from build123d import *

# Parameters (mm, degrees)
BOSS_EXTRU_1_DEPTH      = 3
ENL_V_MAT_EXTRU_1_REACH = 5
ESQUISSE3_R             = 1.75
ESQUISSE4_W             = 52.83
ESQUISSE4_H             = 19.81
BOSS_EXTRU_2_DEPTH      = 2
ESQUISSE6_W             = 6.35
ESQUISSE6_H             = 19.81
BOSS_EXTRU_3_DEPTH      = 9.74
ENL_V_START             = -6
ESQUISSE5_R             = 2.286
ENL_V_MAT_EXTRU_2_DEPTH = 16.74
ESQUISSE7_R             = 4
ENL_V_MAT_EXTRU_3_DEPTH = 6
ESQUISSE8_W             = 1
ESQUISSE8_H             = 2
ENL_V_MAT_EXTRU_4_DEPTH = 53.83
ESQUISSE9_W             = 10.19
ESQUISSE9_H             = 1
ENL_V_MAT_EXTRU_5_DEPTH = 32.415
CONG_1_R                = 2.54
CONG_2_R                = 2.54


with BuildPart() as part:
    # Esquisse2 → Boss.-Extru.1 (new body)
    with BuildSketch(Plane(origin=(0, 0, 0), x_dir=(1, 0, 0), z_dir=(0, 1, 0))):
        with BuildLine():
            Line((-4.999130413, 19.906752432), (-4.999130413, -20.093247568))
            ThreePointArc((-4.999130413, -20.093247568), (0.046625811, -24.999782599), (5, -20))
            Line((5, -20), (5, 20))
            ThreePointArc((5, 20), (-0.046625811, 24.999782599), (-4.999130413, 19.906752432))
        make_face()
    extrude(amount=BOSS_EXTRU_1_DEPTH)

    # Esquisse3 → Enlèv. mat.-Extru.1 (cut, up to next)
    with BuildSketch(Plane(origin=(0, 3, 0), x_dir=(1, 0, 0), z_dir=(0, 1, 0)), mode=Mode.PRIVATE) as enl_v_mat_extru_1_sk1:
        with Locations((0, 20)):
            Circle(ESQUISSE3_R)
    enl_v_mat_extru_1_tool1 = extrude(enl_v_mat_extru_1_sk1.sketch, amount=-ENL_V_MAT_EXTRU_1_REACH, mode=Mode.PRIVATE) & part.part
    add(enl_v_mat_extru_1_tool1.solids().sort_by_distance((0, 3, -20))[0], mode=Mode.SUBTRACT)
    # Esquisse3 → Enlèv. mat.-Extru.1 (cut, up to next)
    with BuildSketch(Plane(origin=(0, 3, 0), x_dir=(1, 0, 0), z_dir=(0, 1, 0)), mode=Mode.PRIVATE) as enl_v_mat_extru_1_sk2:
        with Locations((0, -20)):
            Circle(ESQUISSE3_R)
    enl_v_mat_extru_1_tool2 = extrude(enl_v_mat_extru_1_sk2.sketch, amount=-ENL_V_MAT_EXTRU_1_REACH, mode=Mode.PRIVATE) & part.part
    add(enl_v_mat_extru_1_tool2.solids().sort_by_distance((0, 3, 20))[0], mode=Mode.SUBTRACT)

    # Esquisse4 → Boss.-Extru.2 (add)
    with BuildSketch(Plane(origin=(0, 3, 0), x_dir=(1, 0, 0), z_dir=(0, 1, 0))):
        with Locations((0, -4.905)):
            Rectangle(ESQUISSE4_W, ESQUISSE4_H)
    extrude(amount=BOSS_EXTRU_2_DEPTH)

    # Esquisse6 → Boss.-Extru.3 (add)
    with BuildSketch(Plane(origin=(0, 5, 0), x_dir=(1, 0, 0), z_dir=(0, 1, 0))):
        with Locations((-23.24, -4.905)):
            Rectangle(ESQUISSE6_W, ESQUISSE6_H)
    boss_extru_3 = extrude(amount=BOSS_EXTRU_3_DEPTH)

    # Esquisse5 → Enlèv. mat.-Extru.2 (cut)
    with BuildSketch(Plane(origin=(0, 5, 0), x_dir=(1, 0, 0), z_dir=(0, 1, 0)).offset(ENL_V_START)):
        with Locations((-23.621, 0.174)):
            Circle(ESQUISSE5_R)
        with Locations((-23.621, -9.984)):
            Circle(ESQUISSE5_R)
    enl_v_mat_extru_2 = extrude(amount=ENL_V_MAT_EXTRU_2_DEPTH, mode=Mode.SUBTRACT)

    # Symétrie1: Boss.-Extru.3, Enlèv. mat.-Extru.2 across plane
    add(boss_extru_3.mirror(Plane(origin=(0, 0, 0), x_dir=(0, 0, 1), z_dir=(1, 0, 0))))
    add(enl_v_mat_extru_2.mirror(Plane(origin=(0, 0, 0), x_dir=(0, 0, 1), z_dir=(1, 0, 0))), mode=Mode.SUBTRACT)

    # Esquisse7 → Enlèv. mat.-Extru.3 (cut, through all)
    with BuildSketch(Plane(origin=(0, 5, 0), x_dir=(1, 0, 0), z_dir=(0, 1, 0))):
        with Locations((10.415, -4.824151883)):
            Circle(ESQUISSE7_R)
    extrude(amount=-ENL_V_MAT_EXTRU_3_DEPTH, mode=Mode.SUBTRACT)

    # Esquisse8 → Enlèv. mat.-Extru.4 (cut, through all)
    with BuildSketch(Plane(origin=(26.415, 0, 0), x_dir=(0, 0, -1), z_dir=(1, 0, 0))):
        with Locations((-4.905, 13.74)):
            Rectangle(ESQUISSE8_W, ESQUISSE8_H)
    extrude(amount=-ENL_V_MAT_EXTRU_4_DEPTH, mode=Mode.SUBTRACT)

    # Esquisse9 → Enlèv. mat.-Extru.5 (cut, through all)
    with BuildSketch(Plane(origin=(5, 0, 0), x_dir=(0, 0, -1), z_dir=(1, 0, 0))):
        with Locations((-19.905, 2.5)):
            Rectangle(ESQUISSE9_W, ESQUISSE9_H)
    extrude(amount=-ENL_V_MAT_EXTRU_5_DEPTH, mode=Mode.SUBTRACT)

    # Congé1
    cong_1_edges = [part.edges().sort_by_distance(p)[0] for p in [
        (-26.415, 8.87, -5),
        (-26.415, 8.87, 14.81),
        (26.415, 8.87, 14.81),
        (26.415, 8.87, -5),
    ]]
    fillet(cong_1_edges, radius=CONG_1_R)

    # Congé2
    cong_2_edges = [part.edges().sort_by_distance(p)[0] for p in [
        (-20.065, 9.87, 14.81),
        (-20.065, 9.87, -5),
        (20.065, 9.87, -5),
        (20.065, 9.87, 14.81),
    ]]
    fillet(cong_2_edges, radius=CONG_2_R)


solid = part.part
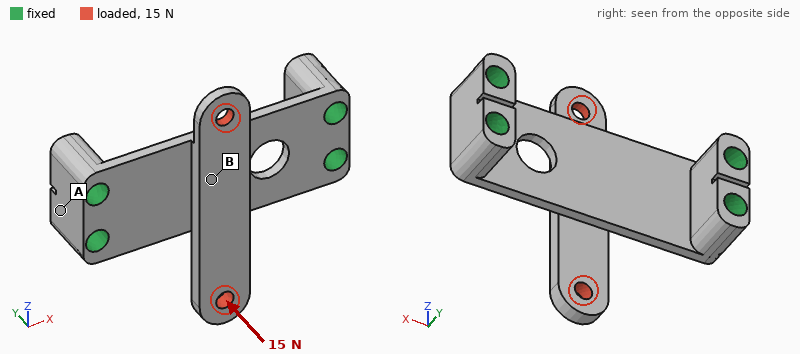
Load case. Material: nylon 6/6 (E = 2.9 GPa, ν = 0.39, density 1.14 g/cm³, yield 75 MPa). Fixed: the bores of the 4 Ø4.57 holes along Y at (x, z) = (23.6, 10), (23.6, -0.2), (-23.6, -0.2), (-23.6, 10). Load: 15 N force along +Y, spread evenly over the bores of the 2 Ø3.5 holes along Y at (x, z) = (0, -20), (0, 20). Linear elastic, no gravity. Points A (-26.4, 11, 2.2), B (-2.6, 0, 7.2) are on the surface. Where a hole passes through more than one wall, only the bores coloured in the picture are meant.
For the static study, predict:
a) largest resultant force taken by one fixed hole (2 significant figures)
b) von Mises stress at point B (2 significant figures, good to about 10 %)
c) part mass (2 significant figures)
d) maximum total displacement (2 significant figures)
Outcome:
13 N
2.2 MPa
5.5 g
0.77 mm
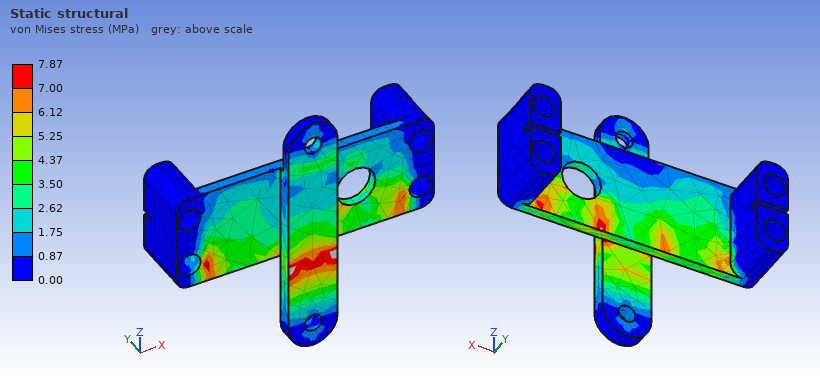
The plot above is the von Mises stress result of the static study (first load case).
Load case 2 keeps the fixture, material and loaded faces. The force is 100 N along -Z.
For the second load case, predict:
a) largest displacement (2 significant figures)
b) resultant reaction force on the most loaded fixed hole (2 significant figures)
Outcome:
0.74 mm
61 N
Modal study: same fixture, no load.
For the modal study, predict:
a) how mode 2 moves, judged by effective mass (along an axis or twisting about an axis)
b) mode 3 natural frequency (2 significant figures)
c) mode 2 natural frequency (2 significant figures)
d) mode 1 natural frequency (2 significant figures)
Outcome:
along Y
3100 Hz
1500 Hz
830 Hz
